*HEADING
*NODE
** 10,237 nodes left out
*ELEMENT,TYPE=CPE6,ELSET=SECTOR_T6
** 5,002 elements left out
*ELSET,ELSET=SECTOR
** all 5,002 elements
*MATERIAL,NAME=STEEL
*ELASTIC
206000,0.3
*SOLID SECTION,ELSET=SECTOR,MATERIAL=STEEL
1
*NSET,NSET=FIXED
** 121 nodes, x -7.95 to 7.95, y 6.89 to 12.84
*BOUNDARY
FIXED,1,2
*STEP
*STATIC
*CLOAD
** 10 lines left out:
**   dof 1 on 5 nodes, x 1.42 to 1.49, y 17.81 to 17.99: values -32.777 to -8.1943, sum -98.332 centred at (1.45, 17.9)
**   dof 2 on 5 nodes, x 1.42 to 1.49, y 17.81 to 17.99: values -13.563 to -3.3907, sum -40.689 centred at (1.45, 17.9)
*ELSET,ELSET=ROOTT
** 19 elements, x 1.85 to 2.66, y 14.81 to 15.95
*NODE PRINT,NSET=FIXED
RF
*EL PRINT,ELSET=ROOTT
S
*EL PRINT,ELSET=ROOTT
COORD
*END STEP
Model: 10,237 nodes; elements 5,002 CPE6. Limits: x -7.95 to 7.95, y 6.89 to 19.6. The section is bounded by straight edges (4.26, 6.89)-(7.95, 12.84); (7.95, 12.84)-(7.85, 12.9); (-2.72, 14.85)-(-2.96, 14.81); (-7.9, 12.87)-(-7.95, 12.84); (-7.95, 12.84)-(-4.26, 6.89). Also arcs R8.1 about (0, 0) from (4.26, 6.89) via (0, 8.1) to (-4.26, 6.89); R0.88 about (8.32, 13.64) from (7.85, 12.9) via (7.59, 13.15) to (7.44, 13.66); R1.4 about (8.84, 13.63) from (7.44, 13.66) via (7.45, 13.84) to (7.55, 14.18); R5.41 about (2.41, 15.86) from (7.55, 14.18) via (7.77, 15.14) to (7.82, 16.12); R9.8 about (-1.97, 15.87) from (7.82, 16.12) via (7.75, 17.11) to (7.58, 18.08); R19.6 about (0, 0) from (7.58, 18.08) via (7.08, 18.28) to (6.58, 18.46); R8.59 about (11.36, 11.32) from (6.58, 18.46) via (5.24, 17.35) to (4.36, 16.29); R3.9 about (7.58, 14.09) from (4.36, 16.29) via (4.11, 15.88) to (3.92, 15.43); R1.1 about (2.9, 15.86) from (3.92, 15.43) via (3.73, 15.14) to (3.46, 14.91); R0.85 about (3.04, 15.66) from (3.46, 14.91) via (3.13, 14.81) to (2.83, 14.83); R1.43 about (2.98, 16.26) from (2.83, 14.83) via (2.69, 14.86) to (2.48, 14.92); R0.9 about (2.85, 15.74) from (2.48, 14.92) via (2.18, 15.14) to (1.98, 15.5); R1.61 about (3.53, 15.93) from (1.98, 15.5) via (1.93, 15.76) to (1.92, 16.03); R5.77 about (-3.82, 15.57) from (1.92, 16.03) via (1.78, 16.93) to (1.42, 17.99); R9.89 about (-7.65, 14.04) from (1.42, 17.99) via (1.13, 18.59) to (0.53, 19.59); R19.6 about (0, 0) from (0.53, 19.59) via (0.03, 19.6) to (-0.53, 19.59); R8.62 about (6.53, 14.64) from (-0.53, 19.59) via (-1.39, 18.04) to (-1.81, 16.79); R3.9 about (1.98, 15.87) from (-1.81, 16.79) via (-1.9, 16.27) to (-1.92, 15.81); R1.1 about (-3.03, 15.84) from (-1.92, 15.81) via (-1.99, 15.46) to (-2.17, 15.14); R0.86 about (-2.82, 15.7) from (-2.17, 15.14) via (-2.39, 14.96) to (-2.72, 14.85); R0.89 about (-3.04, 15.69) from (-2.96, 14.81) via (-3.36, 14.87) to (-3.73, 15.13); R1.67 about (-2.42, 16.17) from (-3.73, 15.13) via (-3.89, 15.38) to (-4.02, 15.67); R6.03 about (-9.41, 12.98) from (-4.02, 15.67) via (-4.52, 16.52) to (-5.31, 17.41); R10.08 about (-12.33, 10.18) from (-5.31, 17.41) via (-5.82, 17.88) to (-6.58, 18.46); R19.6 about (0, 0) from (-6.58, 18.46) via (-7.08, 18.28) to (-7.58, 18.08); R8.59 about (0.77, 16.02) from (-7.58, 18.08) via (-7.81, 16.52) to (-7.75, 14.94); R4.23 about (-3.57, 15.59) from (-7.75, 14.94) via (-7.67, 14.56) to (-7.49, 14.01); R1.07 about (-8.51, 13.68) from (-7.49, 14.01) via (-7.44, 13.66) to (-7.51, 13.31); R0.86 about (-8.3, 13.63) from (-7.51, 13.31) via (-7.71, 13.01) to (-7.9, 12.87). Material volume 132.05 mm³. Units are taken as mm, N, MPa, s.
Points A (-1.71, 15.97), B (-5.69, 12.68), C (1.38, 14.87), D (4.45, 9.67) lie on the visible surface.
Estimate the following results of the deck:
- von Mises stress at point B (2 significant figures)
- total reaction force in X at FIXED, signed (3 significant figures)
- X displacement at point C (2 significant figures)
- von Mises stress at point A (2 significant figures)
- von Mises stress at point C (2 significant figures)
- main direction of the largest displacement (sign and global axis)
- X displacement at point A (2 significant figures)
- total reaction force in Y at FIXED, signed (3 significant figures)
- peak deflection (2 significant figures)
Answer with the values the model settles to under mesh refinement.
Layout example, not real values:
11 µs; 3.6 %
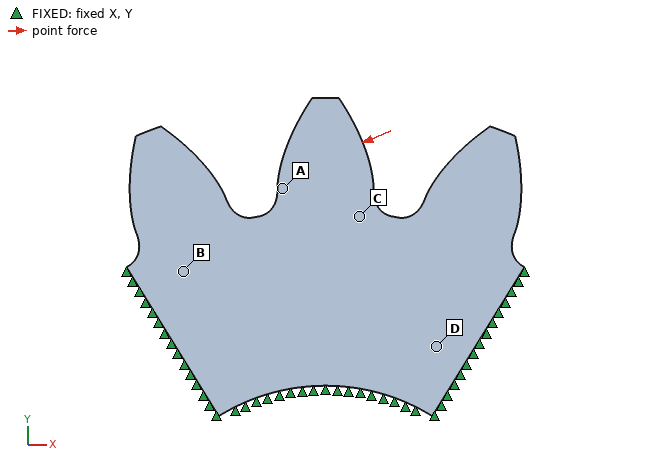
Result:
15 MPa; 98.3 N; -5.5e-04 mm; 61 MPa; 20 MPa; -X; -0.0013 mm; 40.7 N; 0.0037 mm
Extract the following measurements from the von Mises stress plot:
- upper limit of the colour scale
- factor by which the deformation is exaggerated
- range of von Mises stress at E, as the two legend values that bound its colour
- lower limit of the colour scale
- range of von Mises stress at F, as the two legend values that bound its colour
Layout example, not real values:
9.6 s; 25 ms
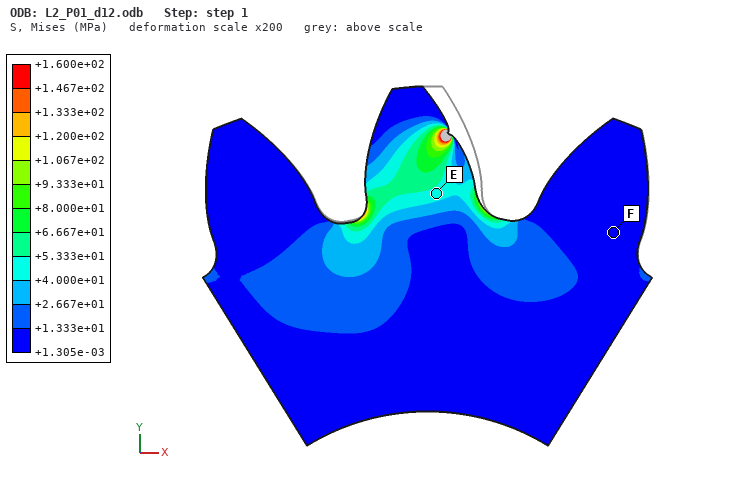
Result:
+1.600e+02 MPa; 200; +4.000e+01 to +5.333e+01 MPa; +1.305e-03 MPa; +1.305e-03 to +1.333e+01 MPa
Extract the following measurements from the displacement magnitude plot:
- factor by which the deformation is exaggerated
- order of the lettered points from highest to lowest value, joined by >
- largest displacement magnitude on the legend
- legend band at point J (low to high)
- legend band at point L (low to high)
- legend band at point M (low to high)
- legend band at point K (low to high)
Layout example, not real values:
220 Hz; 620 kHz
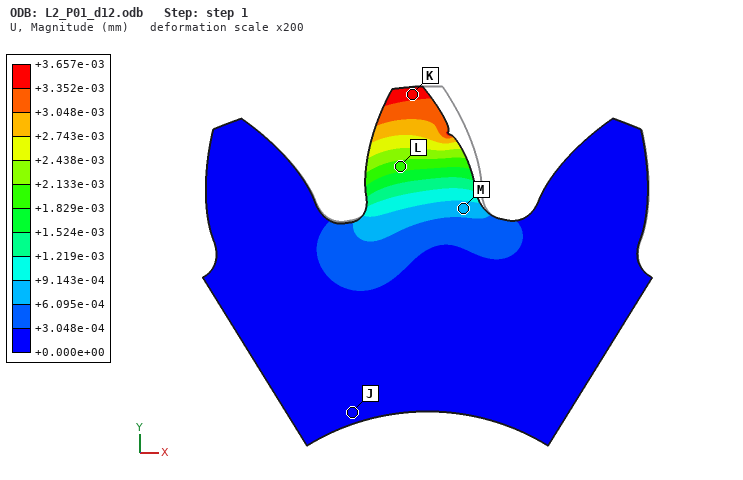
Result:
200; K > L > M > J; +3.657e-03 mm; +0.000e+00 to +3.048e-04 mm; +1.829e-03 to +2.133e-03 mm; +6.095e-04 to +9.143e-04 mm; +3.352e-03 to +3.657e-03 mm
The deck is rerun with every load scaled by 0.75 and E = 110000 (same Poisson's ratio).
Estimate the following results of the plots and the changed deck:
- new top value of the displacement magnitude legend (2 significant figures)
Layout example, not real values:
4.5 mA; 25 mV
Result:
0.0051 mm
